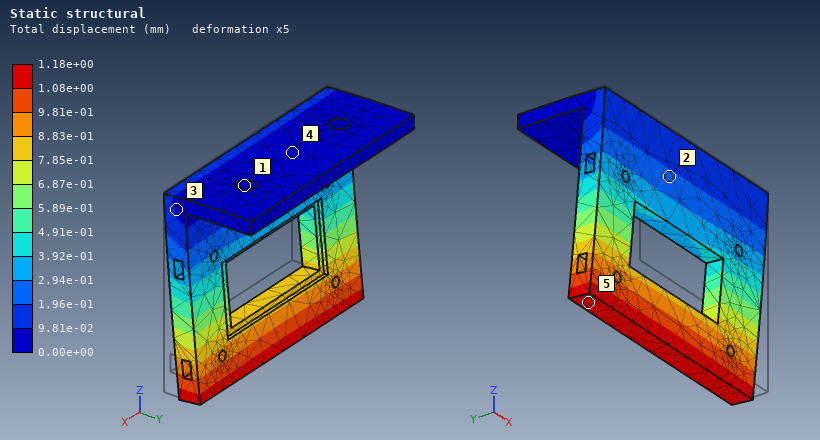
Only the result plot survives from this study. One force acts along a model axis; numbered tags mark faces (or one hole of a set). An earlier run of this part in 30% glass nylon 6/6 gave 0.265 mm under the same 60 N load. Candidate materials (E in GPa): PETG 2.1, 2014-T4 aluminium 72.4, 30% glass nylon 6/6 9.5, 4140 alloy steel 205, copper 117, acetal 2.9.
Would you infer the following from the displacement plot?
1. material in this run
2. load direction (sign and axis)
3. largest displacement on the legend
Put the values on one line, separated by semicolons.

PETG; +Y; 1.18e+00 mm
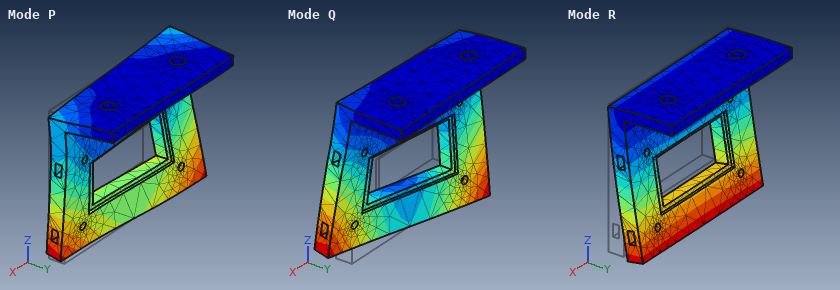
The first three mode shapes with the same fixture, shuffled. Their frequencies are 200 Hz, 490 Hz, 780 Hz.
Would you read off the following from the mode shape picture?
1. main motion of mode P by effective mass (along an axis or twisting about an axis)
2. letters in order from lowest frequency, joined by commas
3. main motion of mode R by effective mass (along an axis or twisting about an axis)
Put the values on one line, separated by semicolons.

along X; R, Q, P; along Y
